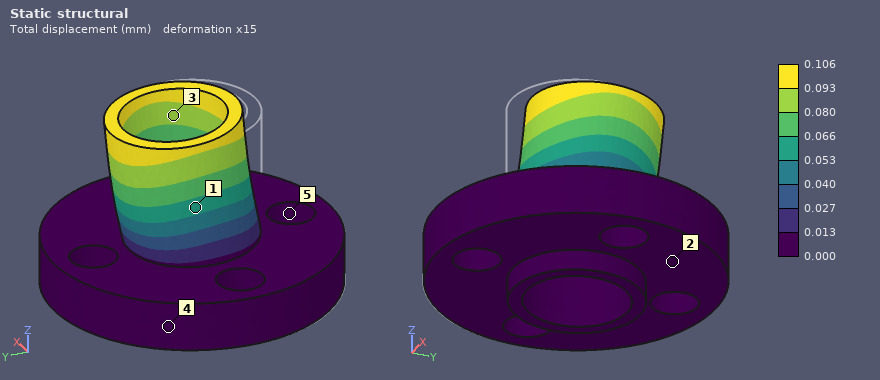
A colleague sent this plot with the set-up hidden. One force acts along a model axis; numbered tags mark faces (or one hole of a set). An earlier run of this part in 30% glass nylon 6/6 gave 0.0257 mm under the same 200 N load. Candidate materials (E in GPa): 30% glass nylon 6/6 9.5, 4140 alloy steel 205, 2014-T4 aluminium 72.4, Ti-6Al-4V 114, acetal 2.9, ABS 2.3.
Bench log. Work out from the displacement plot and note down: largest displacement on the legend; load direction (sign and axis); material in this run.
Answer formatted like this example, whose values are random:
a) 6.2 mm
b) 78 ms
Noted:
a) 0.106 mm
b) +Y
c) ABS
